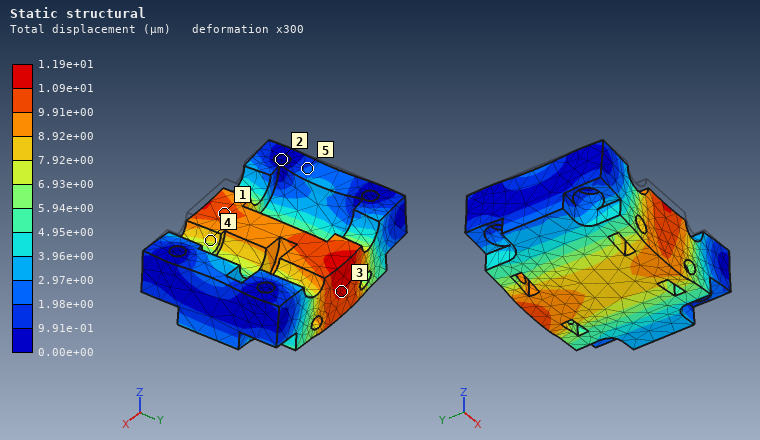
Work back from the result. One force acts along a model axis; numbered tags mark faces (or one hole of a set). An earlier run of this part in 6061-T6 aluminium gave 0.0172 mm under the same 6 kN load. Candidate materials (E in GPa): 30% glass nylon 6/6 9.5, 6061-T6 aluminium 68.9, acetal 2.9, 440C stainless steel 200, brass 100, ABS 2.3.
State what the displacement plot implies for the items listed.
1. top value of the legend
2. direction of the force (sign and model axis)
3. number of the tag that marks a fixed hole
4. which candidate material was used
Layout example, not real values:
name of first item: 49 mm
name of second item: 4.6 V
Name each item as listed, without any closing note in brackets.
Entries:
top value of the legend: 1.19e+01 µm
direction of the force: -Z
number of the tag that marks a fixed hole: 2
which candidate material was used: brass
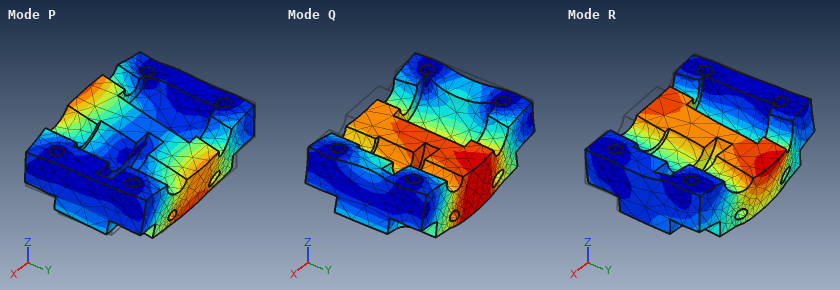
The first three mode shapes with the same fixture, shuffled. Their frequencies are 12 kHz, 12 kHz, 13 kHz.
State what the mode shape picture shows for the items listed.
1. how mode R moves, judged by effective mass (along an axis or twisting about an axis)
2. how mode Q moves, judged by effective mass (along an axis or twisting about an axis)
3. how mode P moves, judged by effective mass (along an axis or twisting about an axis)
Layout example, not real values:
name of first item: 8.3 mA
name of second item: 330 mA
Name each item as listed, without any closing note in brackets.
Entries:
how mode R moves, judged by effective mass: along Y
how mode Q moves, judged by effective mass: along Z
how mode P moves, judged by effective mass: along Y
